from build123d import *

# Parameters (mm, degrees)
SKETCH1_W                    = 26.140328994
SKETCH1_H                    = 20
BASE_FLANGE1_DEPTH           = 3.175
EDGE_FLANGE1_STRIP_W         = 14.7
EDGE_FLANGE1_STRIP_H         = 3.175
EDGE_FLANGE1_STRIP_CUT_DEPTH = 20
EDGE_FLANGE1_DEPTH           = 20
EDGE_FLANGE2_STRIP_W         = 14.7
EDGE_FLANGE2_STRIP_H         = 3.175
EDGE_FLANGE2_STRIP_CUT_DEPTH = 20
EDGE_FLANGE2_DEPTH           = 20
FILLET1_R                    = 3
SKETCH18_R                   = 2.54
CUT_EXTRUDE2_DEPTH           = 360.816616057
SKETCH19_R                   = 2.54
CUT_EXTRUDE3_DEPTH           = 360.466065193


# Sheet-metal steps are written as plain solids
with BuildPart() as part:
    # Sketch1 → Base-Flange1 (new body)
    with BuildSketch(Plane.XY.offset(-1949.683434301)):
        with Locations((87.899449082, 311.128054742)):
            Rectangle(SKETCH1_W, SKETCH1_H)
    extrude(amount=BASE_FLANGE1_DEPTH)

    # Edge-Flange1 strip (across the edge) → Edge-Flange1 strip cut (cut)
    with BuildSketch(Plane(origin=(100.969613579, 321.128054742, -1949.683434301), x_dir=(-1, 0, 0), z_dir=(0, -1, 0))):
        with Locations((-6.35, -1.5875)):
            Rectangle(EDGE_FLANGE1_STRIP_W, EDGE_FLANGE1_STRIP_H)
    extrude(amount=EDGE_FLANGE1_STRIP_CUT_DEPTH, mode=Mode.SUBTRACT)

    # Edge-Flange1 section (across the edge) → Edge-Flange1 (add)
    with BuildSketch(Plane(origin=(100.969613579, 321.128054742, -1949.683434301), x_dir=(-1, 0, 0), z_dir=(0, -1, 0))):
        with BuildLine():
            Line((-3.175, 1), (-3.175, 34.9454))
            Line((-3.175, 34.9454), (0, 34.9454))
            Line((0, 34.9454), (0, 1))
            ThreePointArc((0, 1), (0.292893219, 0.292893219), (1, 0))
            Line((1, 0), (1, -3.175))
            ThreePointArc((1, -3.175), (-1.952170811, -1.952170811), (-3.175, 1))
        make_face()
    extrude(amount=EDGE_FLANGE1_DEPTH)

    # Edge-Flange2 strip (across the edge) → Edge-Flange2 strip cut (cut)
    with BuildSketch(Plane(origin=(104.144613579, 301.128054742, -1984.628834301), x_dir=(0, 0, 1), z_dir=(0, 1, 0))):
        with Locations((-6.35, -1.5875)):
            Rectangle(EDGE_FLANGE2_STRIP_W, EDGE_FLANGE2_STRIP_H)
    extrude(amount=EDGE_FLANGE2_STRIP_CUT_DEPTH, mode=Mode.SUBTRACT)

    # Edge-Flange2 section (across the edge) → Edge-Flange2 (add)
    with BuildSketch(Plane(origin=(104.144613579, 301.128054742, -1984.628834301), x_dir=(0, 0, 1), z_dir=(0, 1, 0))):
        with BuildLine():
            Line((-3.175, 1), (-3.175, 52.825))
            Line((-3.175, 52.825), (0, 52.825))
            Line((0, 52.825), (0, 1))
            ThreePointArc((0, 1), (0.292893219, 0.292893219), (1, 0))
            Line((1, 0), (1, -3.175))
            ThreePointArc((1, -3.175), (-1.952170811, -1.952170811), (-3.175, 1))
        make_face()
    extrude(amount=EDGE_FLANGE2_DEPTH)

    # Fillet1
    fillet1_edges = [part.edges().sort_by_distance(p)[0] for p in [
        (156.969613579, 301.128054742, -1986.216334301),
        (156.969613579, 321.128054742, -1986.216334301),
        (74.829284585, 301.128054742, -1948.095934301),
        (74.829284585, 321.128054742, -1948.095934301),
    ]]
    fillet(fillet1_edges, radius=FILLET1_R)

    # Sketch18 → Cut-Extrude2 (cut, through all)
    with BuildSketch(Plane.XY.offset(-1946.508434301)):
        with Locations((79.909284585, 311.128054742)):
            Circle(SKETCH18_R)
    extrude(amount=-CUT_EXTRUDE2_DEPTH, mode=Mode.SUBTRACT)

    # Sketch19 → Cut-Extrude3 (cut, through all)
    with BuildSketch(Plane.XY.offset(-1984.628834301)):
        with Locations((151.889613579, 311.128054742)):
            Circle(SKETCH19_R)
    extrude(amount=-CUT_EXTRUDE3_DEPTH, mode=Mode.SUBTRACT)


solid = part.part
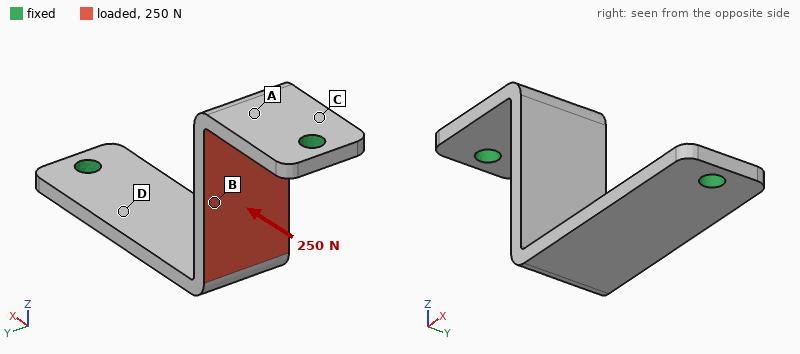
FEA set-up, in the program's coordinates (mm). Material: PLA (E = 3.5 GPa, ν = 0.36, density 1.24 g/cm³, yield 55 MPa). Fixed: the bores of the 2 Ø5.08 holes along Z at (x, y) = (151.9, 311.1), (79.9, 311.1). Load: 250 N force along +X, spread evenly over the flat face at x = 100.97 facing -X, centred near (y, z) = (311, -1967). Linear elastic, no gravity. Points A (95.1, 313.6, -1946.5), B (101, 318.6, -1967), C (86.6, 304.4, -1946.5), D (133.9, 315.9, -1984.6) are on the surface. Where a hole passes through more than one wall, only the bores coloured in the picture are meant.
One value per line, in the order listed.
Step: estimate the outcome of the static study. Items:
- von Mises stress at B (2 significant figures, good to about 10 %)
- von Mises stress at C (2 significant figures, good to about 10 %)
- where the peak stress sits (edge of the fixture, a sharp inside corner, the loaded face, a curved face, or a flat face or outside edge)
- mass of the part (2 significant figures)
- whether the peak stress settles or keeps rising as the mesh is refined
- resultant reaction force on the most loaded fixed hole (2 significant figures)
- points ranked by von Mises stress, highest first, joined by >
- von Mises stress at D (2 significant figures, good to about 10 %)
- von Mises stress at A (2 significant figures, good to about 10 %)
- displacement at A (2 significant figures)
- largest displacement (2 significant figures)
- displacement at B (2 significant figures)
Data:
28 MPa
13 MPa
edge of the fixture
9.1 g
keeps rising
130 N
B > C > A > D
5.5 MPa
9.8 MPa
0.30 mm
0.99 mm
0.96 mm
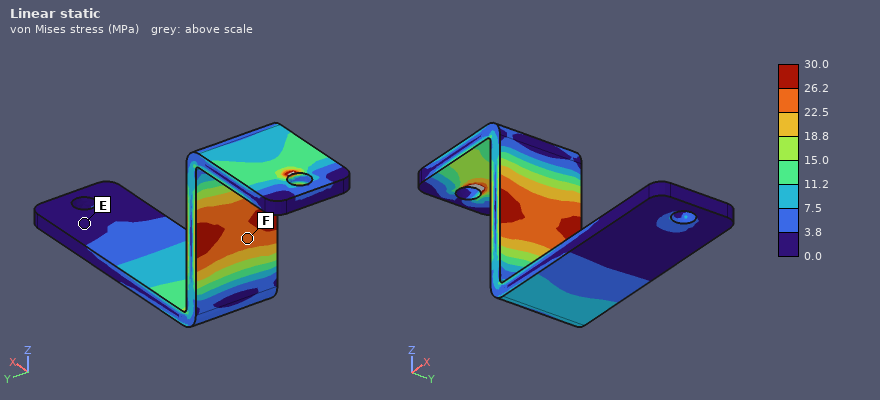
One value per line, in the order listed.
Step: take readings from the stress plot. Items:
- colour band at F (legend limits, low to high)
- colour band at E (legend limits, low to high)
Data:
22.5 to 26.2 MPa
0.0 to 3.8 MPa
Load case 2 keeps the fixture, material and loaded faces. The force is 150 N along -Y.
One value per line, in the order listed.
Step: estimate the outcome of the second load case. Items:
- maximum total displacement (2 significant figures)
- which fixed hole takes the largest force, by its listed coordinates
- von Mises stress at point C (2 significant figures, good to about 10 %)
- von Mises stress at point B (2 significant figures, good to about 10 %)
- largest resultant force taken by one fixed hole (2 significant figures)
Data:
0.87 mm
(79.9, 311.1)
5.5 MPa
5.0 MPa
83 N
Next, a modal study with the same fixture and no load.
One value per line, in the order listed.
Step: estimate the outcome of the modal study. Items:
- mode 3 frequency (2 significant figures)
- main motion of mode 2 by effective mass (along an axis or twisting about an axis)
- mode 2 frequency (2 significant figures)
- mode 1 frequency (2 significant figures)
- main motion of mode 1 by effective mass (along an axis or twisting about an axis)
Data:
1800 Hz
along Y
1000 Hz
790 Hz
along Z
